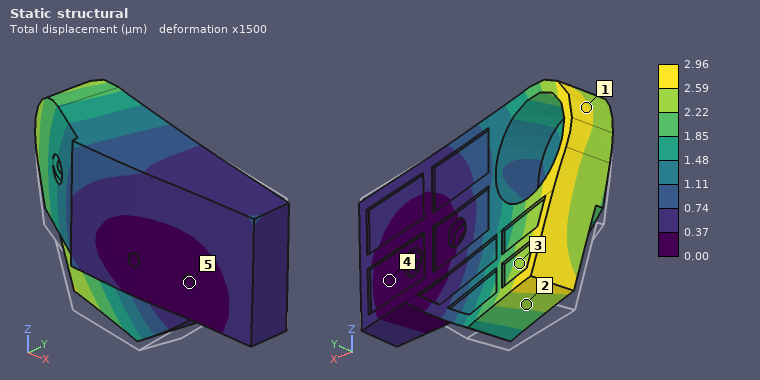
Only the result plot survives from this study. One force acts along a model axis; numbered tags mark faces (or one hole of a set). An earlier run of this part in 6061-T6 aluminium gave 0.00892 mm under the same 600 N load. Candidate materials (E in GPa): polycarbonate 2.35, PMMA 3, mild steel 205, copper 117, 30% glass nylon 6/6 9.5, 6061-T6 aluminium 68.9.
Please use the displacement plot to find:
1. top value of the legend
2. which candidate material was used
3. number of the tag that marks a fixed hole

2.96 µm
mild steel
5
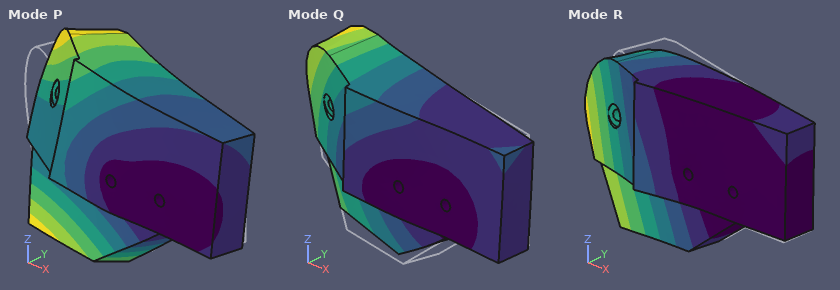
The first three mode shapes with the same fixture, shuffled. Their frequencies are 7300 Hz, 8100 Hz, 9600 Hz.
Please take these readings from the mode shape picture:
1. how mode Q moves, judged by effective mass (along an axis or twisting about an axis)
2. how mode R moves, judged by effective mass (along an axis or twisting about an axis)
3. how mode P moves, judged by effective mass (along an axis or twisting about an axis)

along Z
along Y
twisting about X
